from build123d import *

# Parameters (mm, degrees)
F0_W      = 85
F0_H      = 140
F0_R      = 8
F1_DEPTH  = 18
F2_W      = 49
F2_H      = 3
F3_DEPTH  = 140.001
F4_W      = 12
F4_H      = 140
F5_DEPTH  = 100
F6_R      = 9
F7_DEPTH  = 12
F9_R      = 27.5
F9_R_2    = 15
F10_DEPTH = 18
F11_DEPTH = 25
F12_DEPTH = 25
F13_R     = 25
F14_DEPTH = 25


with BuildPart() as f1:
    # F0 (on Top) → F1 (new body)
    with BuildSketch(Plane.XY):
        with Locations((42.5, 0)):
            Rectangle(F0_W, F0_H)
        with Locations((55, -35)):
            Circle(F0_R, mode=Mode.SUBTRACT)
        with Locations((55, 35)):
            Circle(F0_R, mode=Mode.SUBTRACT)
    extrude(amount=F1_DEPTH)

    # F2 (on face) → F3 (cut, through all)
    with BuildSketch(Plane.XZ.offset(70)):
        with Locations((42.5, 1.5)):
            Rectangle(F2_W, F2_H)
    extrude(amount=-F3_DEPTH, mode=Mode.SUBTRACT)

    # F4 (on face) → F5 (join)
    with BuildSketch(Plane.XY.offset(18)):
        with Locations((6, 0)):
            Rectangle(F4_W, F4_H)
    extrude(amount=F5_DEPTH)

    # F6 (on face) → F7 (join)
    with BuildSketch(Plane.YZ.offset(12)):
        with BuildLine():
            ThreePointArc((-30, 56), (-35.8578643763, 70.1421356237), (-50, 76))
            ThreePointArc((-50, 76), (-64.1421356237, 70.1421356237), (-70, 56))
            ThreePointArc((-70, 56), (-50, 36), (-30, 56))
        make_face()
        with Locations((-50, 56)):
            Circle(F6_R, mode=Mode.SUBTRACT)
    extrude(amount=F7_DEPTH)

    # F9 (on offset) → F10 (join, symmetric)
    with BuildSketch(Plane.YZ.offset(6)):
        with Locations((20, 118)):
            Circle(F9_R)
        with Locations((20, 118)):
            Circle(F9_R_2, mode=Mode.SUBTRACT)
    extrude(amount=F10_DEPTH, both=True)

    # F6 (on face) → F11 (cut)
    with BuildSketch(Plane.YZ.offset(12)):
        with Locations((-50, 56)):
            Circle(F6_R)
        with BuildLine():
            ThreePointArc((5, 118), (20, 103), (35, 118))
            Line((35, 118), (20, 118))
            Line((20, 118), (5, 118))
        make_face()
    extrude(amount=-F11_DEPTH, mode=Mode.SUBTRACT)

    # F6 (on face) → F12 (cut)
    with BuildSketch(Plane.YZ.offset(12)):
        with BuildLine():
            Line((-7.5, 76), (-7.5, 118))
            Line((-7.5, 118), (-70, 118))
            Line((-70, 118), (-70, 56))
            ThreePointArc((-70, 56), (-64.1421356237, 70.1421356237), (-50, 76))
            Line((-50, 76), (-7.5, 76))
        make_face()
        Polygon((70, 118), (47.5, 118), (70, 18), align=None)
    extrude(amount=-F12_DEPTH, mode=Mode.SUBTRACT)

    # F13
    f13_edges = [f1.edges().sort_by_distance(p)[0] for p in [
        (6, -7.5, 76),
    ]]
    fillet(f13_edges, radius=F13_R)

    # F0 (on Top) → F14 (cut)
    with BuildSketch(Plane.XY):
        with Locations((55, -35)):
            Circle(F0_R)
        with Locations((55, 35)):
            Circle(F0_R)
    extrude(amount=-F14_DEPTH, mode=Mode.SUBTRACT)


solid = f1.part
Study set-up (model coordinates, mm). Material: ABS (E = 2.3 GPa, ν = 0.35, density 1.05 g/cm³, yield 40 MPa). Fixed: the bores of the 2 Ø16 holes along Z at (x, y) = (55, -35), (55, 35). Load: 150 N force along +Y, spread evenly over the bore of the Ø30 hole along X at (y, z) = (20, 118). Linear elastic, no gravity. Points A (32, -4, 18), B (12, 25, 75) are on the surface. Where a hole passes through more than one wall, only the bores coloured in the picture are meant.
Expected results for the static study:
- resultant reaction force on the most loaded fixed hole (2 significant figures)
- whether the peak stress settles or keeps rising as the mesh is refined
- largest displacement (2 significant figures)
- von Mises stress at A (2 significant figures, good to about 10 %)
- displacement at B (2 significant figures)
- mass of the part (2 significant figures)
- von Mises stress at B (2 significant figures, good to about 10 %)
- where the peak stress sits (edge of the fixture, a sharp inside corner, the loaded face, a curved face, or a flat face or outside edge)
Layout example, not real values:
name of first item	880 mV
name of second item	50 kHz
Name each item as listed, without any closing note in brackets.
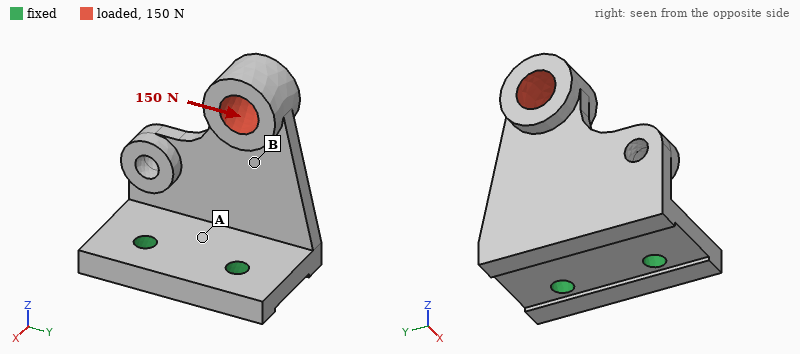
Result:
resultant reaction force on the most loaded fixed hole	210 N
whether the peak stress settles or keeps rising as the mesh is refined	keeps rising
largest displacement	0.36 mm
von Mises stress at A	1.1 MPa
displacement at B	0.17 mm
mass of the part	380 g
von Mises stress at B	0.37 MPa
where the peak stress sits	edge of the fixture
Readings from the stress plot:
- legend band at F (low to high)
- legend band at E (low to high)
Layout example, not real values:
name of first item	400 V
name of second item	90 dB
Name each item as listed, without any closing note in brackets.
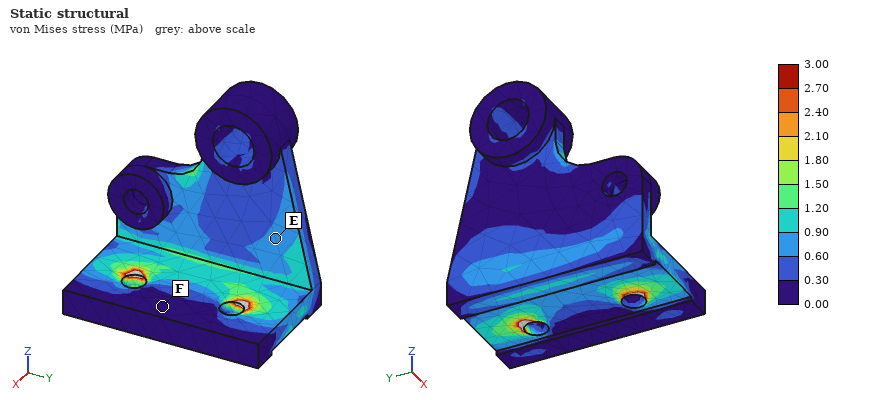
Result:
legend band at F	0.00 to 0.30 MPa
legend band at E	0.60 to 0.90 MPa
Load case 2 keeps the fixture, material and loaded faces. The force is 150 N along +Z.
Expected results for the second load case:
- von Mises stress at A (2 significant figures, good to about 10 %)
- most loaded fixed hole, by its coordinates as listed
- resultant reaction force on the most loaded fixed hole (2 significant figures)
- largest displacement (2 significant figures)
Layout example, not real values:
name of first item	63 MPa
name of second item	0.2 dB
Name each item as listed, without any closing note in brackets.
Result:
von Mises stress at A	0.60 MPa
most loaded fixed hole, by its coordinates as listed	(55, 35)
resultant reaction force on the most loaded fixed hole	110 N
largest displacement	0.28 mm
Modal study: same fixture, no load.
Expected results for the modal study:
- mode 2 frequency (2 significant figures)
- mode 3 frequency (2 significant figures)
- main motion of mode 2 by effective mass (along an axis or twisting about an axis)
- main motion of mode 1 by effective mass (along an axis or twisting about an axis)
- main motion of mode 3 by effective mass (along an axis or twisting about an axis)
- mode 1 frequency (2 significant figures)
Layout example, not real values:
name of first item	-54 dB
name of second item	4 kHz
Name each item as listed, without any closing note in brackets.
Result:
mode 2 frequency	360 Hz
mode 3 frequency	520 Hz
main motion of mode 2 by effective mass	along Y
main motion of mode 1 by effective mass	along X
main motion of mode 3 by effective mass	along Z
mode 1 frequency	140 Hz
